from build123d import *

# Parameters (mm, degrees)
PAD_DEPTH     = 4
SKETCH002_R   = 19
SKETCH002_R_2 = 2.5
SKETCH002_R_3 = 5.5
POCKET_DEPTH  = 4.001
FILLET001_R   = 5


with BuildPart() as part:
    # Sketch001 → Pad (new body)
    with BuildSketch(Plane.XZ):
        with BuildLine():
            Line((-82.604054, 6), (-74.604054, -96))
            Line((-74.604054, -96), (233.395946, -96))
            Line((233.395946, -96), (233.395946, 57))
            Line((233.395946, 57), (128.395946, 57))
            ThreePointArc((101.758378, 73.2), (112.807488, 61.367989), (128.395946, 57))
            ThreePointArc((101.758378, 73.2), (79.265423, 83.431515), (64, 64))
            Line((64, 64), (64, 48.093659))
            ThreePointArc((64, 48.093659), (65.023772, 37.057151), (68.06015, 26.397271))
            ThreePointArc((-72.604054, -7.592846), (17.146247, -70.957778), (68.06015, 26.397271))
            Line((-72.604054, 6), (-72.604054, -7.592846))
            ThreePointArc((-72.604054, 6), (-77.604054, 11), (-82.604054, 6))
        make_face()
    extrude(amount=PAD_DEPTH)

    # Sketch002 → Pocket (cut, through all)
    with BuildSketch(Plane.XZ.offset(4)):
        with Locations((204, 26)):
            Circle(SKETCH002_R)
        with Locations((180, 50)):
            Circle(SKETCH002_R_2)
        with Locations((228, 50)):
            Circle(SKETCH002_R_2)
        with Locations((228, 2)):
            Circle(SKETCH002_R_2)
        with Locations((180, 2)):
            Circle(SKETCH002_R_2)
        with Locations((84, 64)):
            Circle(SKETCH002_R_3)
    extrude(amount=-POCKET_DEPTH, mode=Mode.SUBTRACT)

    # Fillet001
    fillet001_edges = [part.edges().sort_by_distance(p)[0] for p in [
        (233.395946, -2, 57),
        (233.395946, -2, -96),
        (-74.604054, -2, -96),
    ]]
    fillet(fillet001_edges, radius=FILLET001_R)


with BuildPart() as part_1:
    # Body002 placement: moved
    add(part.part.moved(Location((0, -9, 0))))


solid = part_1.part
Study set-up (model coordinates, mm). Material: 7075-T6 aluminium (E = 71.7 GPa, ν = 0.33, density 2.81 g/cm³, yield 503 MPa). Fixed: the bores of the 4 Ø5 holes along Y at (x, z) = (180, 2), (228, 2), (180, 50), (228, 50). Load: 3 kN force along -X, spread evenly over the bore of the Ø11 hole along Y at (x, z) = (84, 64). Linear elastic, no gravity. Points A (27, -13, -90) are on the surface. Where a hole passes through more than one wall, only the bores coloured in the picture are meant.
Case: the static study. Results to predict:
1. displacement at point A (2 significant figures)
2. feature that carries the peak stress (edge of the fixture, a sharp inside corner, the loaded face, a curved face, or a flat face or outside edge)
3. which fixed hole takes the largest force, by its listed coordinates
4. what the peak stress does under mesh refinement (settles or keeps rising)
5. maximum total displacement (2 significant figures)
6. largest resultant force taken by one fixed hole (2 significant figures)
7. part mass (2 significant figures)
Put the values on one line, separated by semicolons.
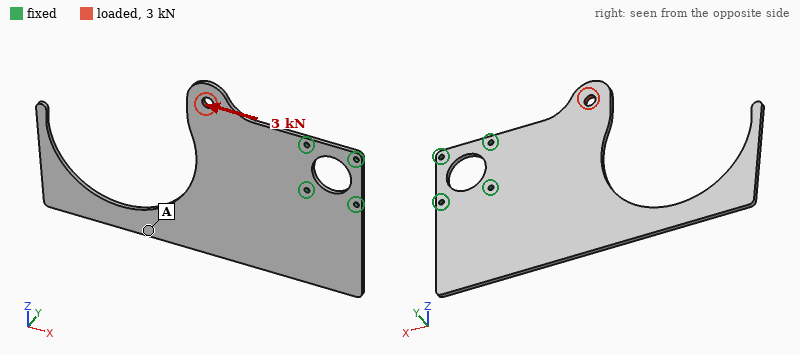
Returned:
58 µm; edge of the fixture; (180, 50); keeps rising; 97 µm; 2.9 kN; 350 g
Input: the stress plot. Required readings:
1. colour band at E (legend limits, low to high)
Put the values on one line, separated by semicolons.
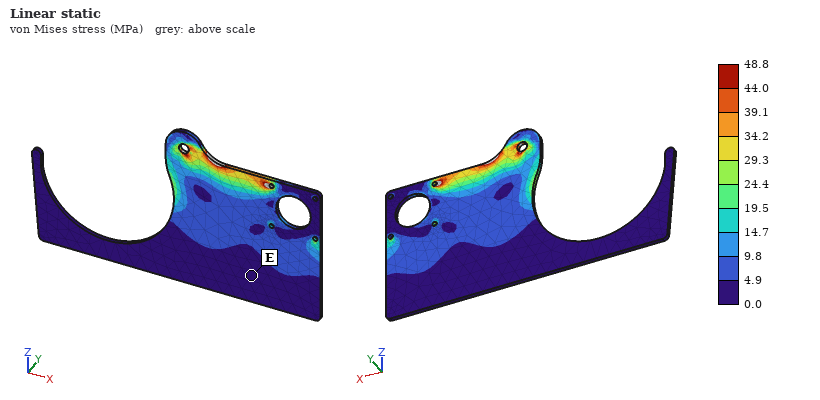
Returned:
0.0 to 4.9 MPa
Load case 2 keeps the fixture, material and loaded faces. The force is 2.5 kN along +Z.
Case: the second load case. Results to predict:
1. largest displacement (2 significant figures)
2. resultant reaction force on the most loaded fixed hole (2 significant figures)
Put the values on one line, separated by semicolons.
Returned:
0.17 mm; 3.5 kN
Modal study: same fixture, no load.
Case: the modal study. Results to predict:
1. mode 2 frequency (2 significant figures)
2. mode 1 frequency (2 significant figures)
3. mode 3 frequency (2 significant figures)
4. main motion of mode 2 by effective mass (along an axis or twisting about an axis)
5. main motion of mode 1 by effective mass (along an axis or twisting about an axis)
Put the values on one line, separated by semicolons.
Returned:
190 Hz; 62 Hz; 270 Hz; along Y; along Y
